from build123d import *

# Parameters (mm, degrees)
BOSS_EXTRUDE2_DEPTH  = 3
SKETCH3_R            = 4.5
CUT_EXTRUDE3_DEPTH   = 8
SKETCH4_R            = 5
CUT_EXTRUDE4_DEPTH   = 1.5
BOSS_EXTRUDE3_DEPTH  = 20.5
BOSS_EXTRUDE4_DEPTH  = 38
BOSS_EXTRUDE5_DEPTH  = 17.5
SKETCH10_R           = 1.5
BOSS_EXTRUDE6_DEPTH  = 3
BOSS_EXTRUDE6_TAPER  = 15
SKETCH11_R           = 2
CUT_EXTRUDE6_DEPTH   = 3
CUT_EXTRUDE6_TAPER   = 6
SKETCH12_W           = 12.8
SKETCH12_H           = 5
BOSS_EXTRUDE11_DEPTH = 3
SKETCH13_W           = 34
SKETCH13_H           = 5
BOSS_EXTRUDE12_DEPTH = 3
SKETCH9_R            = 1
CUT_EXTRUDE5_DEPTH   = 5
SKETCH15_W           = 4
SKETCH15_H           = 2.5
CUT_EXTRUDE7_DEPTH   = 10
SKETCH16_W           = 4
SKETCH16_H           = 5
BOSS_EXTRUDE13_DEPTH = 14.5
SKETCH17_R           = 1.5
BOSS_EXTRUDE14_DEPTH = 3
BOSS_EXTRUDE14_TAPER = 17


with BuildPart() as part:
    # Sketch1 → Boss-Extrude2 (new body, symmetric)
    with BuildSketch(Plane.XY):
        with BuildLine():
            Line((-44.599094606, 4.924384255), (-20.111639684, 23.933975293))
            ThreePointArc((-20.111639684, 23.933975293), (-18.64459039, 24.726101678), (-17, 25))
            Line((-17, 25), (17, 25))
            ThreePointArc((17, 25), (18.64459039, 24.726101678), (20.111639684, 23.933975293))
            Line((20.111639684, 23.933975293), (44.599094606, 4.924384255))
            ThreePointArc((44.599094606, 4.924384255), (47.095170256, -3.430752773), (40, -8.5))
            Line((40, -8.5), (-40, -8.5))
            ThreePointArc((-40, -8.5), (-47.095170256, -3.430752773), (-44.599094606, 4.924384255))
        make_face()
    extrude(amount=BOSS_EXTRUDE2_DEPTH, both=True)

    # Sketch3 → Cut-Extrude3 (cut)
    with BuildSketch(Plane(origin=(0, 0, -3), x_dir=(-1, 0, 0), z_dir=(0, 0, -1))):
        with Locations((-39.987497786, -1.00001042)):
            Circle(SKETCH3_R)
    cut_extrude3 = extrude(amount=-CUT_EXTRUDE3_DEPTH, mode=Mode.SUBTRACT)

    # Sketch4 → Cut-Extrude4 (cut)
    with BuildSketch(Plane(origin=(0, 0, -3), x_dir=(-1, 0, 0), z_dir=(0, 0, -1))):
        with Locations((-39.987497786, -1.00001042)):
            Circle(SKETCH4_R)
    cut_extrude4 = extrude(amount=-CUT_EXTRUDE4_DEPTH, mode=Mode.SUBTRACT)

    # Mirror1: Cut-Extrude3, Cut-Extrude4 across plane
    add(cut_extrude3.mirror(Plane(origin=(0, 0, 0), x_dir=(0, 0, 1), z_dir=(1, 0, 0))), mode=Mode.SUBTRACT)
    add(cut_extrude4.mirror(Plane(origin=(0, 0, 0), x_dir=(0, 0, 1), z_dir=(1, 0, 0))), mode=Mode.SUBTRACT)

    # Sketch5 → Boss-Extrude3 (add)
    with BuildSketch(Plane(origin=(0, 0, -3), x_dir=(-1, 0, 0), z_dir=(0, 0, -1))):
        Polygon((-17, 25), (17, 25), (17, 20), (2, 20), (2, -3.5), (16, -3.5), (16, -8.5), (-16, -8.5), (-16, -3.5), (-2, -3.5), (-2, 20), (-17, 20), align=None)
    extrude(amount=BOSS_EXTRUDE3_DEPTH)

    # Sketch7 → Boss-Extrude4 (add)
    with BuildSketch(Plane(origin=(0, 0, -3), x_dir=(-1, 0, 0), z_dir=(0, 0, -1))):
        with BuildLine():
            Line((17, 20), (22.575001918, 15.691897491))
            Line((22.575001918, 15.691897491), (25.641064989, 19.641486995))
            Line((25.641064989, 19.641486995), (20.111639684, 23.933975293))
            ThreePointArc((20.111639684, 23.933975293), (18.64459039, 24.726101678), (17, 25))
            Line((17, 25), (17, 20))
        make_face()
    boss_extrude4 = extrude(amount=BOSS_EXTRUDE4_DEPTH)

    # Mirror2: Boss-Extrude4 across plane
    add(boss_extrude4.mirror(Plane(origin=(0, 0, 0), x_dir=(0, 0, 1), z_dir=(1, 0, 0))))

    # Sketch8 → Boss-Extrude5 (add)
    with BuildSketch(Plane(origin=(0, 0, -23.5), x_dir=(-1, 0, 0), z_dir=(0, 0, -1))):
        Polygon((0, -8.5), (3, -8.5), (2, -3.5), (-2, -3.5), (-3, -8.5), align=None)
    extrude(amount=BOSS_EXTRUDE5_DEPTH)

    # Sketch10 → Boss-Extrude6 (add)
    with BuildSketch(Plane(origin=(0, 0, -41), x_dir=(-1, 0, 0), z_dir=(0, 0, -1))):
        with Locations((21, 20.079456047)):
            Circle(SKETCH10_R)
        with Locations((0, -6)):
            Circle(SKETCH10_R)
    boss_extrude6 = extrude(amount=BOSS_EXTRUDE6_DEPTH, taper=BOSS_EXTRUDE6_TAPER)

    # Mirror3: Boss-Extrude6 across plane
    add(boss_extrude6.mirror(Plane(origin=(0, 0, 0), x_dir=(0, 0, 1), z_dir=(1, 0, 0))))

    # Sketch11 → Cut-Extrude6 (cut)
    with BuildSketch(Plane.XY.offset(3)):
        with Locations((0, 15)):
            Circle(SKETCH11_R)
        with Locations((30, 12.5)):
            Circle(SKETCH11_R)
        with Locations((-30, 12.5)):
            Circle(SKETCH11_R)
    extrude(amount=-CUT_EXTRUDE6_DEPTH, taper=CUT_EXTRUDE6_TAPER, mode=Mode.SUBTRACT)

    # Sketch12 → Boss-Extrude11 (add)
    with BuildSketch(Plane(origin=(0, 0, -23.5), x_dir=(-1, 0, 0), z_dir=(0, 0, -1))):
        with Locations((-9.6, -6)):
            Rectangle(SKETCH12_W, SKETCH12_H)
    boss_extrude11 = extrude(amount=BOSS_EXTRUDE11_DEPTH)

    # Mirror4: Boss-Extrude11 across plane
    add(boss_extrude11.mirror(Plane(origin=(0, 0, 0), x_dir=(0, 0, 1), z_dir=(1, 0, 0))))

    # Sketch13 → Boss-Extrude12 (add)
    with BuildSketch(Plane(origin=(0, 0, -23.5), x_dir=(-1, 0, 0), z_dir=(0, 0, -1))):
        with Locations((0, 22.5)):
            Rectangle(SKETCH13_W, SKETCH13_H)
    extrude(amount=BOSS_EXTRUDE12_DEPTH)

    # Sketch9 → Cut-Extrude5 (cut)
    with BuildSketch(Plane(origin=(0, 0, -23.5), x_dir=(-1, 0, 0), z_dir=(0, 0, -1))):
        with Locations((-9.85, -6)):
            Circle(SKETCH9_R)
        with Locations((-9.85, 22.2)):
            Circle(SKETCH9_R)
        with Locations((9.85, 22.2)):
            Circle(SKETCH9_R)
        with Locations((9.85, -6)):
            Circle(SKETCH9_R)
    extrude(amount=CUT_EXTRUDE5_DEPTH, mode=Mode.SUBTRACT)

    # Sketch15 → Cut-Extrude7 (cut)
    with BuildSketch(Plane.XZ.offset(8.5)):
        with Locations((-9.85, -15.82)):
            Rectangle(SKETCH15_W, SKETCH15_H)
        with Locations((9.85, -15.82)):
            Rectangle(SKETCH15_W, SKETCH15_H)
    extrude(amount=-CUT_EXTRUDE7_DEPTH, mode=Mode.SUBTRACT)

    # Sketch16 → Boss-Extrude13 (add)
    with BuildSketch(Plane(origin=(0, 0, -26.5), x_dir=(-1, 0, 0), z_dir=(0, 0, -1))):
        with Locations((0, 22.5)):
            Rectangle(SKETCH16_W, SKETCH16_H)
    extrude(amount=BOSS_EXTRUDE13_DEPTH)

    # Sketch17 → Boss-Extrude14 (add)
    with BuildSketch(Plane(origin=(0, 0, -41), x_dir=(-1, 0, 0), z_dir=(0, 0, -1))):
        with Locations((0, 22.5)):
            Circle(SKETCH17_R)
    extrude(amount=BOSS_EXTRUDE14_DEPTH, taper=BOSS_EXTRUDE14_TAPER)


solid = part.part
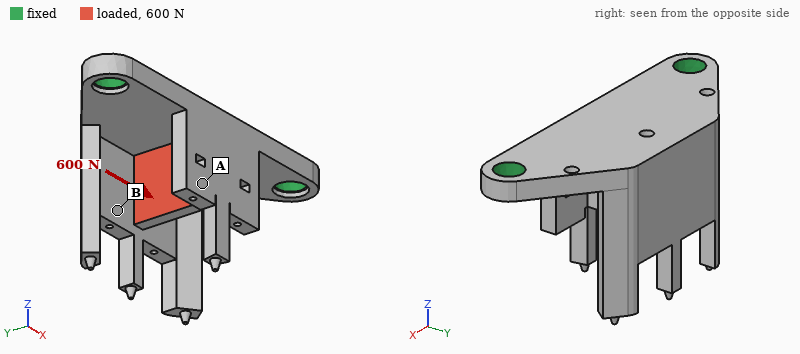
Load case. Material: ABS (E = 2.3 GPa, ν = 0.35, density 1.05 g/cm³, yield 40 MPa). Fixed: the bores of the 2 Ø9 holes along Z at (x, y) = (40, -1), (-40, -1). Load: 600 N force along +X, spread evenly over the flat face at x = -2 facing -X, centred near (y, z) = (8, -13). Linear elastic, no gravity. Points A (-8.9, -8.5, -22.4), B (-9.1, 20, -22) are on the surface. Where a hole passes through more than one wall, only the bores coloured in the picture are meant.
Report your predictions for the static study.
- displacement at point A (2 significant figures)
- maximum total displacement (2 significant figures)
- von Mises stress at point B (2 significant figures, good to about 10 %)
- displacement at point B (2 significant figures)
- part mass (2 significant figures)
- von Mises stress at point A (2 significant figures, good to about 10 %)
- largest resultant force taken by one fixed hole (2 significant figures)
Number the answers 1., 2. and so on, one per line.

1. 0.26 mm
2. 0.63 mm
3. 4.7 MPa
4. 0.29 mm
5. 29 g
6. 1.8 MPa
7. 340 N
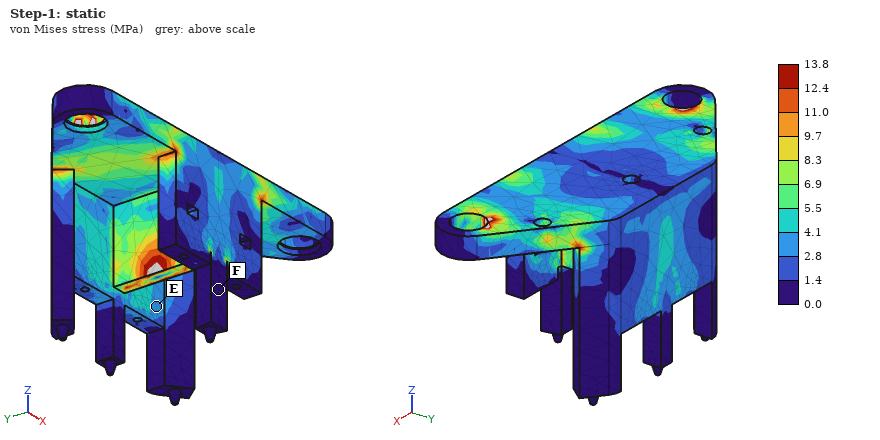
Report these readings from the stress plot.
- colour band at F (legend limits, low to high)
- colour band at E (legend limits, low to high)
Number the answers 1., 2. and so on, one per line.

1. 0.0 to 1.4 MPa
2. 2.8 to 4.1 MPa
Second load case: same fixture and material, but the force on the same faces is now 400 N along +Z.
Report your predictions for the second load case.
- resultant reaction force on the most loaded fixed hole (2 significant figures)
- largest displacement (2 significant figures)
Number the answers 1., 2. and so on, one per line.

1. 230 N
2. 1.2 mm
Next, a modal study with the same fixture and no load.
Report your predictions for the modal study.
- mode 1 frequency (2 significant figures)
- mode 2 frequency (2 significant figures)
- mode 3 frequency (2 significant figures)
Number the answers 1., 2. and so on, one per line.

1. 520 Hz
2. 1200 Hz
3. 1200 Hz
